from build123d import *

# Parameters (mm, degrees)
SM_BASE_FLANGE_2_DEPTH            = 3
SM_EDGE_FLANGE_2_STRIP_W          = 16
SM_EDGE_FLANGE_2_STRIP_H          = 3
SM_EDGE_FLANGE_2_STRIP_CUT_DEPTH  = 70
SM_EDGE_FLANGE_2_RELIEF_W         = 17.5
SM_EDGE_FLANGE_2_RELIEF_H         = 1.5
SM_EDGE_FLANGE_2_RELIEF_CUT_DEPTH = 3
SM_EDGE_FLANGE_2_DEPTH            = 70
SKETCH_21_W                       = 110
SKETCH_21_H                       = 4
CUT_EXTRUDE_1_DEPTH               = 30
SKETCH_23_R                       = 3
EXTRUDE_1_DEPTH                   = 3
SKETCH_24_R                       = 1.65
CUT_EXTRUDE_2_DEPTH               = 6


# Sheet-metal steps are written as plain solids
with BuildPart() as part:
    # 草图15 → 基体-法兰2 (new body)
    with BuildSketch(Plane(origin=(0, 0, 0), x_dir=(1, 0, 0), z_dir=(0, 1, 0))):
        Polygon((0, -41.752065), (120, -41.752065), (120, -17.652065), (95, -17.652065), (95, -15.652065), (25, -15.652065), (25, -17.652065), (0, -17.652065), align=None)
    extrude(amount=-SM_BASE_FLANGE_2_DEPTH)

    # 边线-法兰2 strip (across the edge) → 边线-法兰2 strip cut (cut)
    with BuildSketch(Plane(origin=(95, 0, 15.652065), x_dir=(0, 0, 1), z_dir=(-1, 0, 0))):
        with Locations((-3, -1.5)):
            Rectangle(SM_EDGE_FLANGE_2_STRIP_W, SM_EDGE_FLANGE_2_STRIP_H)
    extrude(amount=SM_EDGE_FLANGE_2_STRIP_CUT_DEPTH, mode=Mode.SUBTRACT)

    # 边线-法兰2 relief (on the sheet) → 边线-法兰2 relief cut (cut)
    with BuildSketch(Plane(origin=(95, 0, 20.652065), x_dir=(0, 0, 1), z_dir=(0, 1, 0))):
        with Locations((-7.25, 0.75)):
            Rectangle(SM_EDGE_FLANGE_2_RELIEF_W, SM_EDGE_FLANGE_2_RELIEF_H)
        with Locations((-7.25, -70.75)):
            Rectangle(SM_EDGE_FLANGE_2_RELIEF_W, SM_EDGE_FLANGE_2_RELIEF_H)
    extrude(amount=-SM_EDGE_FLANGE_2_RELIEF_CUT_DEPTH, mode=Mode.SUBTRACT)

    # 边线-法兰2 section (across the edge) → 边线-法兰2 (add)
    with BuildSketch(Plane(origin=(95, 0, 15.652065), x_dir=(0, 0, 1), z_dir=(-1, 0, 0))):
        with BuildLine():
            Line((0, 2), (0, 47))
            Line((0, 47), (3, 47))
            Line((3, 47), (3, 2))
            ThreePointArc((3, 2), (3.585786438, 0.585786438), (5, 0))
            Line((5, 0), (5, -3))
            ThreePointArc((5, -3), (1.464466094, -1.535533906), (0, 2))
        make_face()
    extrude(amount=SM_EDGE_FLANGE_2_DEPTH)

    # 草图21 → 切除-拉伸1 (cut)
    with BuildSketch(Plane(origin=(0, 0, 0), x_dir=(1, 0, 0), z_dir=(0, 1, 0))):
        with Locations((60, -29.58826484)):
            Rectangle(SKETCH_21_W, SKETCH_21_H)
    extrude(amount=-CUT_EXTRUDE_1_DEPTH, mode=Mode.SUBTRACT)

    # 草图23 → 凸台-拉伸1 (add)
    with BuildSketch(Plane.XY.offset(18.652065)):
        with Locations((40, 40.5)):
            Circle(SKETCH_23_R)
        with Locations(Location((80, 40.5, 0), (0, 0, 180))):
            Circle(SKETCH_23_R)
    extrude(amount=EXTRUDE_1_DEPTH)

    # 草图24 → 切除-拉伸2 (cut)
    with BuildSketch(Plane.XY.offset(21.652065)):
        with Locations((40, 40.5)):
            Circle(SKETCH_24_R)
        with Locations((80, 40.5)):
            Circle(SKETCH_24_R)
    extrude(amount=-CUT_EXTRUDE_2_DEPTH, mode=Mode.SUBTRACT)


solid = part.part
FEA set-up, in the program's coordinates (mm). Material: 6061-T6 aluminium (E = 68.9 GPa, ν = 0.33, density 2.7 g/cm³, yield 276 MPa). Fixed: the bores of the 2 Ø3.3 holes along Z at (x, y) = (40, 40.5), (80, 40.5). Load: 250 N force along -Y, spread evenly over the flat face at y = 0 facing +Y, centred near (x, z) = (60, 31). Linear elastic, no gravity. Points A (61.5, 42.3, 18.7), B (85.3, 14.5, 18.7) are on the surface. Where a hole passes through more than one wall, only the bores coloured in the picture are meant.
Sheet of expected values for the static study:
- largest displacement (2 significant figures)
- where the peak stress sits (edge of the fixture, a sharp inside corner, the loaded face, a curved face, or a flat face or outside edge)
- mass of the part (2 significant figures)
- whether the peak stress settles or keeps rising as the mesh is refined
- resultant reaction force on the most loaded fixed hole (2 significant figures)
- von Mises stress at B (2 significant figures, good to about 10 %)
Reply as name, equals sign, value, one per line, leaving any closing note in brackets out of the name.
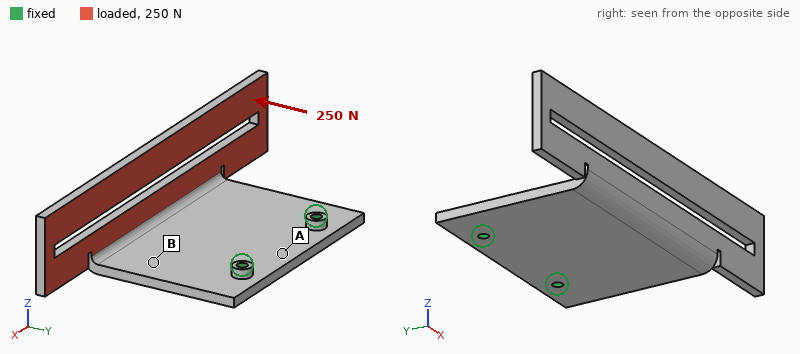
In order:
largest displacement = 1.5 mm
where the peak stress sits = a sharp inside corner
mass of the part = 47 g
whether the peak stress settles or keeps rising as the mesh is refined = keeps rising
resultant reaction force on the most loaded fixed hole = 130 N
von Mises stress at B = 36 MPa
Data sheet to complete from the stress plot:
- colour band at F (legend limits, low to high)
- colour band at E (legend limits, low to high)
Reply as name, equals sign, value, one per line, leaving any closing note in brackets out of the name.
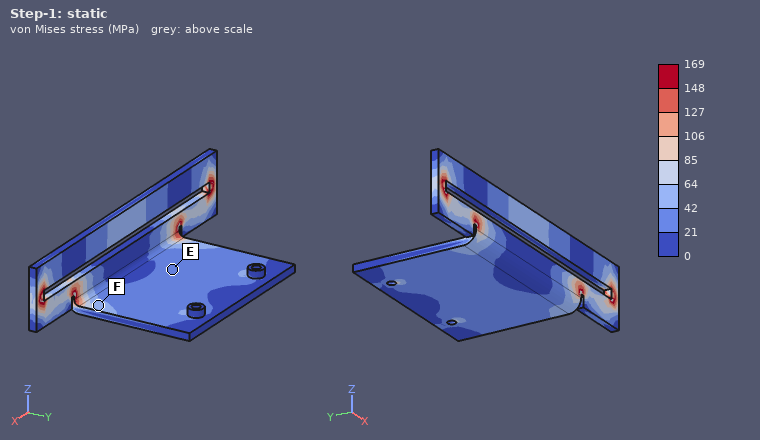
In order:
colour band at F = 42 to 64 MPa
colour band at E = 21 to 42 MPa
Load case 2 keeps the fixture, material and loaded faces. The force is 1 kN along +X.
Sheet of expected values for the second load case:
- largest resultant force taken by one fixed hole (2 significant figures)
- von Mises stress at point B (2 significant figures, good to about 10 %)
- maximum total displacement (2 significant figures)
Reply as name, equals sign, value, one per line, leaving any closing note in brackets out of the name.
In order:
largest resultant force taken by one fixed hole = 1.1 kN
von Mises stress at point B = 78 MPa
maximum total displacement = 1.5 mm
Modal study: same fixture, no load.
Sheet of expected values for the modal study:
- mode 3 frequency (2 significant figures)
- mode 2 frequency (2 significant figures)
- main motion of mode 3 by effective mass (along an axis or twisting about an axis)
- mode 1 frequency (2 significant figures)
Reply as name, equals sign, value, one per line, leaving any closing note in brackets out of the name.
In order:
mode 3 frequency = 760 Hz
mode 2 frequency = 710 Hz
main motion of mode 3 by effective mass = along Z
mode 1 frequency = 510 Hz
